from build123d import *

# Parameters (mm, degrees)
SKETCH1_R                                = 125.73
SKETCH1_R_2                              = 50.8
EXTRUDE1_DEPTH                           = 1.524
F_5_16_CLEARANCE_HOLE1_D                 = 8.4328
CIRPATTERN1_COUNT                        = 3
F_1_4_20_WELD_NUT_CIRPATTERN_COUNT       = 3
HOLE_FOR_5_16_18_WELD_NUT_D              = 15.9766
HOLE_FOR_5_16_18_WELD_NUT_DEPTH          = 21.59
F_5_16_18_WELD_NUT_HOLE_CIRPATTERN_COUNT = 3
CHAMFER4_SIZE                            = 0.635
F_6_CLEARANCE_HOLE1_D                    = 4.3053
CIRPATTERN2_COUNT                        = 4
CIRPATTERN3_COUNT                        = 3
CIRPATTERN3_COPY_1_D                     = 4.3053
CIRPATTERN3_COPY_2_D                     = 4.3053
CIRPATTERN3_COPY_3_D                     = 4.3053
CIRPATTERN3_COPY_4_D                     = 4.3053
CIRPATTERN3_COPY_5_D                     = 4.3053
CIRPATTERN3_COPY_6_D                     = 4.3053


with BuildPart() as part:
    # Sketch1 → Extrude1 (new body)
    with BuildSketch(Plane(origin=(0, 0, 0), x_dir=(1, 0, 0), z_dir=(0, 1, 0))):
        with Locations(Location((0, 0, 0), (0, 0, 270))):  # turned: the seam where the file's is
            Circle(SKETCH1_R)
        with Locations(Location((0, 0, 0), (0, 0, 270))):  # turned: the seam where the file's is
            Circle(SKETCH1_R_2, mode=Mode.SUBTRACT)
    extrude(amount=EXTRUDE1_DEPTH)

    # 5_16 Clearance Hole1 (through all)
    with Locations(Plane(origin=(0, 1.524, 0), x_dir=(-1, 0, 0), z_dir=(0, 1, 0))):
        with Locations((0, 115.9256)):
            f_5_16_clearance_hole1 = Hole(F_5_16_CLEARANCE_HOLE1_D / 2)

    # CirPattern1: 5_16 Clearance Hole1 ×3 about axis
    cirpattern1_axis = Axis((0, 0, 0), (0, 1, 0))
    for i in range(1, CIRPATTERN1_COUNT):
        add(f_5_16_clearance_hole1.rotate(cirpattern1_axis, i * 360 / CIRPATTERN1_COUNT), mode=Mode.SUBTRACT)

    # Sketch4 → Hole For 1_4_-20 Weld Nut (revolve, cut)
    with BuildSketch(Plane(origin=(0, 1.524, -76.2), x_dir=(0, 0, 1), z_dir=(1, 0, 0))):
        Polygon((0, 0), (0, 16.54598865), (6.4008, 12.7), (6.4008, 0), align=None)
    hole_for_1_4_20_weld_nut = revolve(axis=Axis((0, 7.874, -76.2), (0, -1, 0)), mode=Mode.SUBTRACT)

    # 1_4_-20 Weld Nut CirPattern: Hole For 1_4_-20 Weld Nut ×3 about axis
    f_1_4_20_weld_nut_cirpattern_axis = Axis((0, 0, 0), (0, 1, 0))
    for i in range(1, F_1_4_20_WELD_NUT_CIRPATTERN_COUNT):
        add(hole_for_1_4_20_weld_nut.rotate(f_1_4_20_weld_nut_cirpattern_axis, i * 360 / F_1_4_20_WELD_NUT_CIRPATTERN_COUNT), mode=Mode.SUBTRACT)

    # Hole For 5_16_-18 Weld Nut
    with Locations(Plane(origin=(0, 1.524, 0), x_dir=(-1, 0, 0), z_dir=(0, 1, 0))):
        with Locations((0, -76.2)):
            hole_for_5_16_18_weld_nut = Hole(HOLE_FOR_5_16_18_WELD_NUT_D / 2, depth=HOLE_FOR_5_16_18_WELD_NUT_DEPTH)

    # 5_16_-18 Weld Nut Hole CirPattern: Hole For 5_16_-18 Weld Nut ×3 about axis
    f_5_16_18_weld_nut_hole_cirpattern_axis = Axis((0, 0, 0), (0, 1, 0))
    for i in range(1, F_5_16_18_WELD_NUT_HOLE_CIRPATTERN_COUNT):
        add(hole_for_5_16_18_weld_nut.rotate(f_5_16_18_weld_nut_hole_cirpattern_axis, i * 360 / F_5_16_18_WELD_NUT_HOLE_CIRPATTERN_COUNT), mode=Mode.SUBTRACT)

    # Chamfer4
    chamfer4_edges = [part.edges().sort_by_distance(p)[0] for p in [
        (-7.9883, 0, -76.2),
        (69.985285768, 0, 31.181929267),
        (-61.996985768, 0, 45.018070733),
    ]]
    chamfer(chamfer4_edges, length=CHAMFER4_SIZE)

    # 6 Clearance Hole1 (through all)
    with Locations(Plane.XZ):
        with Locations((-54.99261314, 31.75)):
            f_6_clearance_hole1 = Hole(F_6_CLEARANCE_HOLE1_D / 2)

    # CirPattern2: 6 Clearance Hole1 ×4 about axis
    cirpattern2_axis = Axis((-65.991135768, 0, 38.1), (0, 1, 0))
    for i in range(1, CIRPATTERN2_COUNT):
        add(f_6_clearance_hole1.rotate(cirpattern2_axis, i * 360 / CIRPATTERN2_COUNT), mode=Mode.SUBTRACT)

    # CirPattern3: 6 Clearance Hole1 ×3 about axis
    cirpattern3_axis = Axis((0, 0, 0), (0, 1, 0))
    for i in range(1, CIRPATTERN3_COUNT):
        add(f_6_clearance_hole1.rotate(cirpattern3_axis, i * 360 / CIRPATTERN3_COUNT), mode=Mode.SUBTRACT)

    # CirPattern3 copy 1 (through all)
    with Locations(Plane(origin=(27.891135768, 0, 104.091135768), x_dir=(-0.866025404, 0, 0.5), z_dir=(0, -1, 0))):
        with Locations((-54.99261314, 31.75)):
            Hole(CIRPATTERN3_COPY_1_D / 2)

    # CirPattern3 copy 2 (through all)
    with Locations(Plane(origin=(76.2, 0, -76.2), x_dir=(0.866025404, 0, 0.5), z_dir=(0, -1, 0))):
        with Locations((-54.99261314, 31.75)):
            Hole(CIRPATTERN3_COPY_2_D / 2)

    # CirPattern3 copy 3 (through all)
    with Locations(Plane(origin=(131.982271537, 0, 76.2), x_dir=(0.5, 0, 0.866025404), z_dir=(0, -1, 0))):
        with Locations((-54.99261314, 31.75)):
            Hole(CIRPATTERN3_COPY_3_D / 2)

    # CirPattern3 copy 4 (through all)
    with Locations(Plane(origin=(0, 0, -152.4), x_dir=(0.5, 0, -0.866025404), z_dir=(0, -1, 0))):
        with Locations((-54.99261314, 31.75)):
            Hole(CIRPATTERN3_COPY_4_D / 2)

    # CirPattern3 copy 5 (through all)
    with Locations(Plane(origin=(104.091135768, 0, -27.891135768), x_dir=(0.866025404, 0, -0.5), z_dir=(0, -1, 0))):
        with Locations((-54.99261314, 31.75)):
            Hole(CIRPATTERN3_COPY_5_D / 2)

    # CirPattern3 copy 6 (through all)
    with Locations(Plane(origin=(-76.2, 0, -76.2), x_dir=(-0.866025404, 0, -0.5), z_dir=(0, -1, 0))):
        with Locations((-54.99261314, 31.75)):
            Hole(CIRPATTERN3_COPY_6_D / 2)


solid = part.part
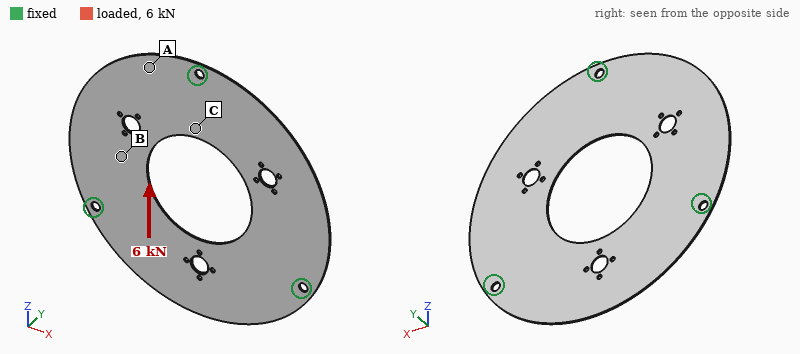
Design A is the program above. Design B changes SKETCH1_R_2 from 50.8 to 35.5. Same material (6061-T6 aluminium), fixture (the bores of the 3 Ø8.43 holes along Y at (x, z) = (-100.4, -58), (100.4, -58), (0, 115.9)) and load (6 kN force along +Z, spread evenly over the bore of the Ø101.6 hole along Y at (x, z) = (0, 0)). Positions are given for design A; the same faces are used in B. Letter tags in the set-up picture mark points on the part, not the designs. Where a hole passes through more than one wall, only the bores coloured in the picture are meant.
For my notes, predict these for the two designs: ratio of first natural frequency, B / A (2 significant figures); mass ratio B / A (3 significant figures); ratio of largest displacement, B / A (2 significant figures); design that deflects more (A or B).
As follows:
1.0
1.10
0.92
A
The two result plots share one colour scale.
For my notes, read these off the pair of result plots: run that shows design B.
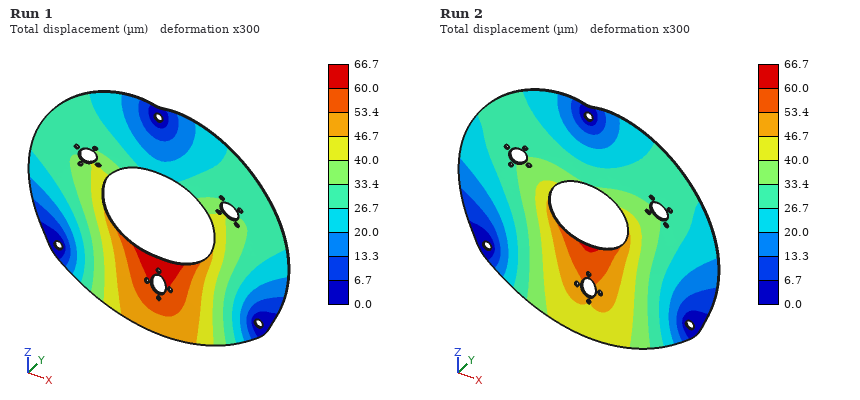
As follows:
Run 2
